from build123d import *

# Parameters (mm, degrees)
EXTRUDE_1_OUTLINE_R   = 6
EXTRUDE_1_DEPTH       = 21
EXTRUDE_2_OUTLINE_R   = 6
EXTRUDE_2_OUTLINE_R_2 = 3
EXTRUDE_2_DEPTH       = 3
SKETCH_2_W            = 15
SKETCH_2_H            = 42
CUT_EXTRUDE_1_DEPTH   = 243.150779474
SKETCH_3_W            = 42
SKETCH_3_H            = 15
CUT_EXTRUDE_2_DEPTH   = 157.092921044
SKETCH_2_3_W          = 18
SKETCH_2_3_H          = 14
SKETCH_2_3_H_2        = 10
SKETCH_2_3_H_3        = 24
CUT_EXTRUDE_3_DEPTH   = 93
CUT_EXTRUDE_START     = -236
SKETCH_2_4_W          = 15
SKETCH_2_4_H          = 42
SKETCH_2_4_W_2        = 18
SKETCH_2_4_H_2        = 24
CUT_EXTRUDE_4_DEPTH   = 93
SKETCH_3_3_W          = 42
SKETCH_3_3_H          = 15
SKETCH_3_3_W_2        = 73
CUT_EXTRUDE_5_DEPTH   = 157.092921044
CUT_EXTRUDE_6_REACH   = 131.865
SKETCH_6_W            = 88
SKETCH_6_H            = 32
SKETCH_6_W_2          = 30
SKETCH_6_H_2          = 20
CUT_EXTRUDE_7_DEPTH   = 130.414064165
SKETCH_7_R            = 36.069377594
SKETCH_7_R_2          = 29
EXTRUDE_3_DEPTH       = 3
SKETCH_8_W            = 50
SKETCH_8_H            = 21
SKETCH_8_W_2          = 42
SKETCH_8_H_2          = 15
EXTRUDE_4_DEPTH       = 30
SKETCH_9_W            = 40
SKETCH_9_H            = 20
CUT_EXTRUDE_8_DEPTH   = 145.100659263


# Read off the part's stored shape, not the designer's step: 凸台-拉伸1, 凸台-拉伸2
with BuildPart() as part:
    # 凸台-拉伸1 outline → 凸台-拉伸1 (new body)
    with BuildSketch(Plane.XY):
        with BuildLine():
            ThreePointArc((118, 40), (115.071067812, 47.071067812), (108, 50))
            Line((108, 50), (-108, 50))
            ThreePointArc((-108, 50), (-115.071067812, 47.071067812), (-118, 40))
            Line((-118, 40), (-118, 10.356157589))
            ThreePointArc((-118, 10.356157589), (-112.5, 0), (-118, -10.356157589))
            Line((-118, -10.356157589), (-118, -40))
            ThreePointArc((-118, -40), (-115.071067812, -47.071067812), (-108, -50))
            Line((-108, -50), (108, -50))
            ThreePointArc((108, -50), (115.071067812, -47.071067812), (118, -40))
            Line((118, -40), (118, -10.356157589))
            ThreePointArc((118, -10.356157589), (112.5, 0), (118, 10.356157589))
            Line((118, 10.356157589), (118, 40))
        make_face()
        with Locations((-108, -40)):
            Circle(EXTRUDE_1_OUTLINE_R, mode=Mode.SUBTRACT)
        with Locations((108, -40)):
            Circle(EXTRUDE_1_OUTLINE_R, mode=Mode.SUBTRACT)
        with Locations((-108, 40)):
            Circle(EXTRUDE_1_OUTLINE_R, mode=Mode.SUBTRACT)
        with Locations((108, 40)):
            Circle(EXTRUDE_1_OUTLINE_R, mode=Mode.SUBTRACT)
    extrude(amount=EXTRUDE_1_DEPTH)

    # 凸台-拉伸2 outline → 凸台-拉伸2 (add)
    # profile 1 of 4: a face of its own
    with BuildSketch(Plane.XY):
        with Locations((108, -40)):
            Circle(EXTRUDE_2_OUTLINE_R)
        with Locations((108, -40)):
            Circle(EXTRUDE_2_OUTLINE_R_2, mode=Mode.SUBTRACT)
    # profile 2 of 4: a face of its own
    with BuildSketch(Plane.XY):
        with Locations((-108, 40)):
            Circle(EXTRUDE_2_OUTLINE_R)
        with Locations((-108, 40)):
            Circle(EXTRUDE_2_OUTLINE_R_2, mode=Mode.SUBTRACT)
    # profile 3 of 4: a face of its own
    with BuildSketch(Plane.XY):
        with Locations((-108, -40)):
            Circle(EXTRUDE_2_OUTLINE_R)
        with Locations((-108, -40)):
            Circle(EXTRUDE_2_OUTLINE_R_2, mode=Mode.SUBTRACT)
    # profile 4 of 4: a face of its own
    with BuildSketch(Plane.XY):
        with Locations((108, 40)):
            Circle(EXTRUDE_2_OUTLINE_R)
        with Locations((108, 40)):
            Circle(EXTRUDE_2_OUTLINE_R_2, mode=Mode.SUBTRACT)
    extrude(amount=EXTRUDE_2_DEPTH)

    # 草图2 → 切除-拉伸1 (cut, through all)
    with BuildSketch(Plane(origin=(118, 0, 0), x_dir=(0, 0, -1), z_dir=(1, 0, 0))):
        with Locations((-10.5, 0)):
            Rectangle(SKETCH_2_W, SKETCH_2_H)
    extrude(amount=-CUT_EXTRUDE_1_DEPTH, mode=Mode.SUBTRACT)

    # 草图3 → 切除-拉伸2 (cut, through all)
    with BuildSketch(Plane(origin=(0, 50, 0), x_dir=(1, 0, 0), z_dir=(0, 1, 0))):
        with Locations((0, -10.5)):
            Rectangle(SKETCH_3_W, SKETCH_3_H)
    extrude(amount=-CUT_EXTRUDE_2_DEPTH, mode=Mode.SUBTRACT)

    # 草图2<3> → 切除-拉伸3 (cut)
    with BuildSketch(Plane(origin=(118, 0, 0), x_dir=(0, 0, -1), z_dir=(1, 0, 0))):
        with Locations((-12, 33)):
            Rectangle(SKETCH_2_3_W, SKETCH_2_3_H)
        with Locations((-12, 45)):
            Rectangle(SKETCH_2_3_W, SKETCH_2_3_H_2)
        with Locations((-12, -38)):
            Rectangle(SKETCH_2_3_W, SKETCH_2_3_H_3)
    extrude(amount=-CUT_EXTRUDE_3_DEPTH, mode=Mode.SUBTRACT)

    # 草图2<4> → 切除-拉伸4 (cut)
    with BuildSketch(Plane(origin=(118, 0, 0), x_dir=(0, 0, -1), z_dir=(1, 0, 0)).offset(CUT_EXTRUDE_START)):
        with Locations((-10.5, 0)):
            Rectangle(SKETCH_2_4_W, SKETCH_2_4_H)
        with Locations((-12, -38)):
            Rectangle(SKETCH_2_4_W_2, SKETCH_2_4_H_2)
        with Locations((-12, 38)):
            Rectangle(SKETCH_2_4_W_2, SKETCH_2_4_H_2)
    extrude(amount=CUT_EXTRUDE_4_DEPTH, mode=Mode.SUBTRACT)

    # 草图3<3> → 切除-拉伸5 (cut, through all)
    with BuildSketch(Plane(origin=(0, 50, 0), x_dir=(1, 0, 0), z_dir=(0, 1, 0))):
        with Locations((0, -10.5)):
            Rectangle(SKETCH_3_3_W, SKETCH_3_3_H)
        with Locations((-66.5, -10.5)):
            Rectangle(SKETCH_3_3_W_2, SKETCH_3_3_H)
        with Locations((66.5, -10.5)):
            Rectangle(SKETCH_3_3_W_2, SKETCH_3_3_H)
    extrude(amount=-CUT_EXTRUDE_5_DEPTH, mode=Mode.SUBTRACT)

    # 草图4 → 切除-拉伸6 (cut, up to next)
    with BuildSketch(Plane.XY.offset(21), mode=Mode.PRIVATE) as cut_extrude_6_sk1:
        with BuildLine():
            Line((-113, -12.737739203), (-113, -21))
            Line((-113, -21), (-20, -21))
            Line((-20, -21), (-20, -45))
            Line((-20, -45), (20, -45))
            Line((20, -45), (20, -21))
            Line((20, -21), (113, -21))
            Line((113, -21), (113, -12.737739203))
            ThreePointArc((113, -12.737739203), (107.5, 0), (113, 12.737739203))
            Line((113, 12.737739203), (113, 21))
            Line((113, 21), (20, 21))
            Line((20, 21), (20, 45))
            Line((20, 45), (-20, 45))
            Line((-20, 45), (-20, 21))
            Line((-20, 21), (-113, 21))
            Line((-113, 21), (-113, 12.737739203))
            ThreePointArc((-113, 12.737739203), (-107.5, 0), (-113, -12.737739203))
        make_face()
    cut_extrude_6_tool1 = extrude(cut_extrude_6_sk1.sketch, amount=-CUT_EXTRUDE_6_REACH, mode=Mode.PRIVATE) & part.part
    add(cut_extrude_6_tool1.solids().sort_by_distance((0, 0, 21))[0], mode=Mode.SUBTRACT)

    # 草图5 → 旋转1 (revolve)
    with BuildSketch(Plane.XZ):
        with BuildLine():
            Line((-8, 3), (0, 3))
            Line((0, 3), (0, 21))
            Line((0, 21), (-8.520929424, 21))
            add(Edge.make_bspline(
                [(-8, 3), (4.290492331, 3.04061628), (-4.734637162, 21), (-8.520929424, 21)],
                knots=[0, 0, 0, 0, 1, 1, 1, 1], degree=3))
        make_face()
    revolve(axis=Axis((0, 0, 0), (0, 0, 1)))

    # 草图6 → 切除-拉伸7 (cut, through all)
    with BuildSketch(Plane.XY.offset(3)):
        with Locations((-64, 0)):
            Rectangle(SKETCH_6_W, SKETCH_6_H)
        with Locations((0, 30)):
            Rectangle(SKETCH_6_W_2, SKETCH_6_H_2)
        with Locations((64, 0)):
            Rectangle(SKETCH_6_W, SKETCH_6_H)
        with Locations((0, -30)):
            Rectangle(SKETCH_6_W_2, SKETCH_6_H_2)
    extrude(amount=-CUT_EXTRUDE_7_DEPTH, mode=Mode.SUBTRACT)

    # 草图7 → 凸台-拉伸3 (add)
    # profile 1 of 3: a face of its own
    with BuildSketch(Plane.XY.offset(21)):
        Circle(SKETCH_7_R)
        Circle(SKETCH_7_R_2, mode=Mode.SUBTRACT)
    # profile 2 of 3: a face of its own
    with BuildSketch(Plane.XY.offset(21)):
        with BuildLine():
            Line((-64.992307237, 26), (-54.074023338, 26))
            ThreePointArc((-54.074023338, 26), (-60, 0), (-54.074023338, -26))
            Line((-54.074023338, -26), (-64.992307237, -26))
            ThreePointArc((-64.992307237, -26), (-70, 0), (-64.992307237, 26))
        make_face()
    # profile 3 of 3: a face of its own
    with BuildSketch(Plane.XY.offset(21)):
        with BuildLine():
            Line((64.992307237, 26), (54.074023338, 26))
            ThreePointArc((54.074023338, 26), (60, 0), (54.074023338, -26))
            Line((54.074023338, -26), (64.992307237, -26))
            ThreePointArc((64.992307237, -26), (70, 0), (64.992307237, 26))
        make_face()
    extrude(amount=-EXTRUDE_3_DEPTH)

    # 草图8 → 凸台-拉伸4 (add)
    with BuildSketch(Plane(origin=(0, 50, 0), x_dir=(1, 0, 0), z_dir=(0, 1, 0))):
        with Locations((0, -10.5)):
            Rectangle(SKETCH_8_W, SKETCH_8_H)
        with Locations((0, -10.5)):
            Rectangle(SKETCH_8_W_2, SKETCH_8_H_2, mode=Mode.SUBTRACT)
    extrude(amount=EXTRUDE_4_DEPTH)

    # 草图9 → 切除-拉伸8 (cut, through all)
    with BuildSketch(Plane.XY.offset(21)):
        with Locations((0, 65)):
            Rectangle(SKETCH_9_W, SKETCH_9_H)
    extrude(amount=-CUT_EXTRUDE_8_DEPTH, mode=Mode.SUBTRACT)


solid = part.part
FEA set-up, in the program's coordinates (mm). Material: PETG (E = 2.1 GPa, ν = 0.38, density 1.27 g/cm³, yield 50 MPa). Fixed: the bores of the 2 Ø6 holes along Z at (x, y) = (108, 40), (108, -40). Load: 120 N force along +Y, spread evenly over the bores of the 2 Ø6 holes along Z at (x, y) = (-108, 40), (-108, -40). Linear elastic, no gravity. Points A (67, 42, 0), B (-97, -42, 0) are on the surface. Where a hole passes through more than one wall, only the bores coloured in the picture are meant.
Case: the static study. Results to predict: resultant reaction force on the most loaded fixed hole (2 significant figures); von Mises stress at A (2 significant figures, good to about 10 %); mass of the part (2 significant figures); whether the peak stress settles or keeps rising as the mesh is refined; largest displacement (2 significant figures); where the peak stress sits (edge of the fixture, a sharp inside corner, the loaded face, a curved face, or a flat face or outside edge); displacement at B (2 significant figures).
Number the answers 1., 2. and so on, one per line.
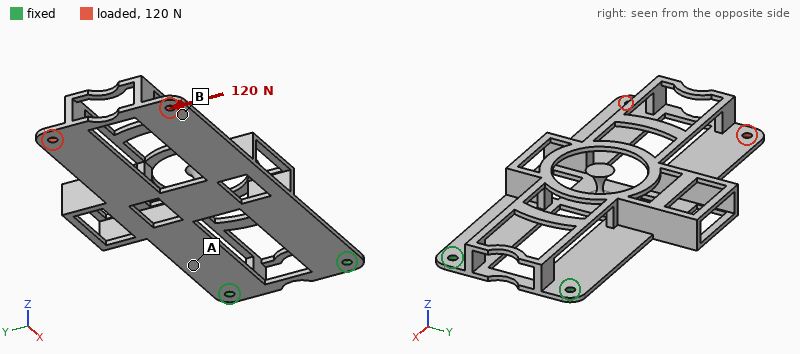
1. 300 N
2. 4.2 MPa
3. 110 g
4. keeps rising
5. 2.7 mm
6. edge of the fixture
7. 2.3 mm
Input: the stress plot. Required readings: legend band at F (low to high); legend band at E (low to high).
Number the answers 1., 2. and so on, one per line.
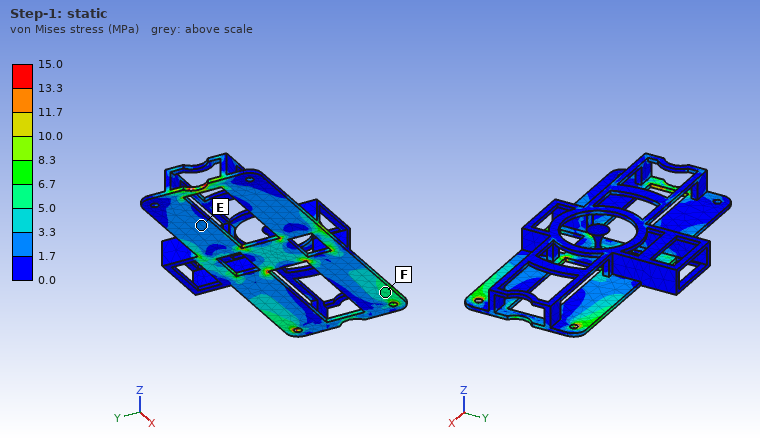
1. 5.0 to 6.7 MPa
2. 1.7 to 3.3 MPa
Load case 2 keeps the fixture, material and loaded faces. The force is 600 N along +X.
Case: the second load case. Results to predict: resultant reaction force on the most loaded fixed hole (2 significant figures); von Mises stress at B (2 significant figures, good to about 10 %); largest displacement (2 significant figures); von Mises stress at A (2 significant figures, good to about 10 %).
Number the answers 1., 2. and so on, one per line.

1. 300 N
2. 5.2 MPa
3. 1.9 mm
4. 3.8 MPa
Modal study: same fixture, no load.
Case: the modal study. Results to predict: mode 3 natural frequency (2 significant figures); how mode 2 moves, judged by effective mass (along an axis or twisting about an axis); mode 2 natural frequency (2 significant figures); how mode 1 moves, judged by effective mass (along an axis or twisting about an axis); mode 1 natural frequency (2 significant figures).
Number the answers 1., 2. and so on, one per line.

1. 110 Hz
2. twisting about X
3. 58 Hz
4. along Z
5. 21 Hz
